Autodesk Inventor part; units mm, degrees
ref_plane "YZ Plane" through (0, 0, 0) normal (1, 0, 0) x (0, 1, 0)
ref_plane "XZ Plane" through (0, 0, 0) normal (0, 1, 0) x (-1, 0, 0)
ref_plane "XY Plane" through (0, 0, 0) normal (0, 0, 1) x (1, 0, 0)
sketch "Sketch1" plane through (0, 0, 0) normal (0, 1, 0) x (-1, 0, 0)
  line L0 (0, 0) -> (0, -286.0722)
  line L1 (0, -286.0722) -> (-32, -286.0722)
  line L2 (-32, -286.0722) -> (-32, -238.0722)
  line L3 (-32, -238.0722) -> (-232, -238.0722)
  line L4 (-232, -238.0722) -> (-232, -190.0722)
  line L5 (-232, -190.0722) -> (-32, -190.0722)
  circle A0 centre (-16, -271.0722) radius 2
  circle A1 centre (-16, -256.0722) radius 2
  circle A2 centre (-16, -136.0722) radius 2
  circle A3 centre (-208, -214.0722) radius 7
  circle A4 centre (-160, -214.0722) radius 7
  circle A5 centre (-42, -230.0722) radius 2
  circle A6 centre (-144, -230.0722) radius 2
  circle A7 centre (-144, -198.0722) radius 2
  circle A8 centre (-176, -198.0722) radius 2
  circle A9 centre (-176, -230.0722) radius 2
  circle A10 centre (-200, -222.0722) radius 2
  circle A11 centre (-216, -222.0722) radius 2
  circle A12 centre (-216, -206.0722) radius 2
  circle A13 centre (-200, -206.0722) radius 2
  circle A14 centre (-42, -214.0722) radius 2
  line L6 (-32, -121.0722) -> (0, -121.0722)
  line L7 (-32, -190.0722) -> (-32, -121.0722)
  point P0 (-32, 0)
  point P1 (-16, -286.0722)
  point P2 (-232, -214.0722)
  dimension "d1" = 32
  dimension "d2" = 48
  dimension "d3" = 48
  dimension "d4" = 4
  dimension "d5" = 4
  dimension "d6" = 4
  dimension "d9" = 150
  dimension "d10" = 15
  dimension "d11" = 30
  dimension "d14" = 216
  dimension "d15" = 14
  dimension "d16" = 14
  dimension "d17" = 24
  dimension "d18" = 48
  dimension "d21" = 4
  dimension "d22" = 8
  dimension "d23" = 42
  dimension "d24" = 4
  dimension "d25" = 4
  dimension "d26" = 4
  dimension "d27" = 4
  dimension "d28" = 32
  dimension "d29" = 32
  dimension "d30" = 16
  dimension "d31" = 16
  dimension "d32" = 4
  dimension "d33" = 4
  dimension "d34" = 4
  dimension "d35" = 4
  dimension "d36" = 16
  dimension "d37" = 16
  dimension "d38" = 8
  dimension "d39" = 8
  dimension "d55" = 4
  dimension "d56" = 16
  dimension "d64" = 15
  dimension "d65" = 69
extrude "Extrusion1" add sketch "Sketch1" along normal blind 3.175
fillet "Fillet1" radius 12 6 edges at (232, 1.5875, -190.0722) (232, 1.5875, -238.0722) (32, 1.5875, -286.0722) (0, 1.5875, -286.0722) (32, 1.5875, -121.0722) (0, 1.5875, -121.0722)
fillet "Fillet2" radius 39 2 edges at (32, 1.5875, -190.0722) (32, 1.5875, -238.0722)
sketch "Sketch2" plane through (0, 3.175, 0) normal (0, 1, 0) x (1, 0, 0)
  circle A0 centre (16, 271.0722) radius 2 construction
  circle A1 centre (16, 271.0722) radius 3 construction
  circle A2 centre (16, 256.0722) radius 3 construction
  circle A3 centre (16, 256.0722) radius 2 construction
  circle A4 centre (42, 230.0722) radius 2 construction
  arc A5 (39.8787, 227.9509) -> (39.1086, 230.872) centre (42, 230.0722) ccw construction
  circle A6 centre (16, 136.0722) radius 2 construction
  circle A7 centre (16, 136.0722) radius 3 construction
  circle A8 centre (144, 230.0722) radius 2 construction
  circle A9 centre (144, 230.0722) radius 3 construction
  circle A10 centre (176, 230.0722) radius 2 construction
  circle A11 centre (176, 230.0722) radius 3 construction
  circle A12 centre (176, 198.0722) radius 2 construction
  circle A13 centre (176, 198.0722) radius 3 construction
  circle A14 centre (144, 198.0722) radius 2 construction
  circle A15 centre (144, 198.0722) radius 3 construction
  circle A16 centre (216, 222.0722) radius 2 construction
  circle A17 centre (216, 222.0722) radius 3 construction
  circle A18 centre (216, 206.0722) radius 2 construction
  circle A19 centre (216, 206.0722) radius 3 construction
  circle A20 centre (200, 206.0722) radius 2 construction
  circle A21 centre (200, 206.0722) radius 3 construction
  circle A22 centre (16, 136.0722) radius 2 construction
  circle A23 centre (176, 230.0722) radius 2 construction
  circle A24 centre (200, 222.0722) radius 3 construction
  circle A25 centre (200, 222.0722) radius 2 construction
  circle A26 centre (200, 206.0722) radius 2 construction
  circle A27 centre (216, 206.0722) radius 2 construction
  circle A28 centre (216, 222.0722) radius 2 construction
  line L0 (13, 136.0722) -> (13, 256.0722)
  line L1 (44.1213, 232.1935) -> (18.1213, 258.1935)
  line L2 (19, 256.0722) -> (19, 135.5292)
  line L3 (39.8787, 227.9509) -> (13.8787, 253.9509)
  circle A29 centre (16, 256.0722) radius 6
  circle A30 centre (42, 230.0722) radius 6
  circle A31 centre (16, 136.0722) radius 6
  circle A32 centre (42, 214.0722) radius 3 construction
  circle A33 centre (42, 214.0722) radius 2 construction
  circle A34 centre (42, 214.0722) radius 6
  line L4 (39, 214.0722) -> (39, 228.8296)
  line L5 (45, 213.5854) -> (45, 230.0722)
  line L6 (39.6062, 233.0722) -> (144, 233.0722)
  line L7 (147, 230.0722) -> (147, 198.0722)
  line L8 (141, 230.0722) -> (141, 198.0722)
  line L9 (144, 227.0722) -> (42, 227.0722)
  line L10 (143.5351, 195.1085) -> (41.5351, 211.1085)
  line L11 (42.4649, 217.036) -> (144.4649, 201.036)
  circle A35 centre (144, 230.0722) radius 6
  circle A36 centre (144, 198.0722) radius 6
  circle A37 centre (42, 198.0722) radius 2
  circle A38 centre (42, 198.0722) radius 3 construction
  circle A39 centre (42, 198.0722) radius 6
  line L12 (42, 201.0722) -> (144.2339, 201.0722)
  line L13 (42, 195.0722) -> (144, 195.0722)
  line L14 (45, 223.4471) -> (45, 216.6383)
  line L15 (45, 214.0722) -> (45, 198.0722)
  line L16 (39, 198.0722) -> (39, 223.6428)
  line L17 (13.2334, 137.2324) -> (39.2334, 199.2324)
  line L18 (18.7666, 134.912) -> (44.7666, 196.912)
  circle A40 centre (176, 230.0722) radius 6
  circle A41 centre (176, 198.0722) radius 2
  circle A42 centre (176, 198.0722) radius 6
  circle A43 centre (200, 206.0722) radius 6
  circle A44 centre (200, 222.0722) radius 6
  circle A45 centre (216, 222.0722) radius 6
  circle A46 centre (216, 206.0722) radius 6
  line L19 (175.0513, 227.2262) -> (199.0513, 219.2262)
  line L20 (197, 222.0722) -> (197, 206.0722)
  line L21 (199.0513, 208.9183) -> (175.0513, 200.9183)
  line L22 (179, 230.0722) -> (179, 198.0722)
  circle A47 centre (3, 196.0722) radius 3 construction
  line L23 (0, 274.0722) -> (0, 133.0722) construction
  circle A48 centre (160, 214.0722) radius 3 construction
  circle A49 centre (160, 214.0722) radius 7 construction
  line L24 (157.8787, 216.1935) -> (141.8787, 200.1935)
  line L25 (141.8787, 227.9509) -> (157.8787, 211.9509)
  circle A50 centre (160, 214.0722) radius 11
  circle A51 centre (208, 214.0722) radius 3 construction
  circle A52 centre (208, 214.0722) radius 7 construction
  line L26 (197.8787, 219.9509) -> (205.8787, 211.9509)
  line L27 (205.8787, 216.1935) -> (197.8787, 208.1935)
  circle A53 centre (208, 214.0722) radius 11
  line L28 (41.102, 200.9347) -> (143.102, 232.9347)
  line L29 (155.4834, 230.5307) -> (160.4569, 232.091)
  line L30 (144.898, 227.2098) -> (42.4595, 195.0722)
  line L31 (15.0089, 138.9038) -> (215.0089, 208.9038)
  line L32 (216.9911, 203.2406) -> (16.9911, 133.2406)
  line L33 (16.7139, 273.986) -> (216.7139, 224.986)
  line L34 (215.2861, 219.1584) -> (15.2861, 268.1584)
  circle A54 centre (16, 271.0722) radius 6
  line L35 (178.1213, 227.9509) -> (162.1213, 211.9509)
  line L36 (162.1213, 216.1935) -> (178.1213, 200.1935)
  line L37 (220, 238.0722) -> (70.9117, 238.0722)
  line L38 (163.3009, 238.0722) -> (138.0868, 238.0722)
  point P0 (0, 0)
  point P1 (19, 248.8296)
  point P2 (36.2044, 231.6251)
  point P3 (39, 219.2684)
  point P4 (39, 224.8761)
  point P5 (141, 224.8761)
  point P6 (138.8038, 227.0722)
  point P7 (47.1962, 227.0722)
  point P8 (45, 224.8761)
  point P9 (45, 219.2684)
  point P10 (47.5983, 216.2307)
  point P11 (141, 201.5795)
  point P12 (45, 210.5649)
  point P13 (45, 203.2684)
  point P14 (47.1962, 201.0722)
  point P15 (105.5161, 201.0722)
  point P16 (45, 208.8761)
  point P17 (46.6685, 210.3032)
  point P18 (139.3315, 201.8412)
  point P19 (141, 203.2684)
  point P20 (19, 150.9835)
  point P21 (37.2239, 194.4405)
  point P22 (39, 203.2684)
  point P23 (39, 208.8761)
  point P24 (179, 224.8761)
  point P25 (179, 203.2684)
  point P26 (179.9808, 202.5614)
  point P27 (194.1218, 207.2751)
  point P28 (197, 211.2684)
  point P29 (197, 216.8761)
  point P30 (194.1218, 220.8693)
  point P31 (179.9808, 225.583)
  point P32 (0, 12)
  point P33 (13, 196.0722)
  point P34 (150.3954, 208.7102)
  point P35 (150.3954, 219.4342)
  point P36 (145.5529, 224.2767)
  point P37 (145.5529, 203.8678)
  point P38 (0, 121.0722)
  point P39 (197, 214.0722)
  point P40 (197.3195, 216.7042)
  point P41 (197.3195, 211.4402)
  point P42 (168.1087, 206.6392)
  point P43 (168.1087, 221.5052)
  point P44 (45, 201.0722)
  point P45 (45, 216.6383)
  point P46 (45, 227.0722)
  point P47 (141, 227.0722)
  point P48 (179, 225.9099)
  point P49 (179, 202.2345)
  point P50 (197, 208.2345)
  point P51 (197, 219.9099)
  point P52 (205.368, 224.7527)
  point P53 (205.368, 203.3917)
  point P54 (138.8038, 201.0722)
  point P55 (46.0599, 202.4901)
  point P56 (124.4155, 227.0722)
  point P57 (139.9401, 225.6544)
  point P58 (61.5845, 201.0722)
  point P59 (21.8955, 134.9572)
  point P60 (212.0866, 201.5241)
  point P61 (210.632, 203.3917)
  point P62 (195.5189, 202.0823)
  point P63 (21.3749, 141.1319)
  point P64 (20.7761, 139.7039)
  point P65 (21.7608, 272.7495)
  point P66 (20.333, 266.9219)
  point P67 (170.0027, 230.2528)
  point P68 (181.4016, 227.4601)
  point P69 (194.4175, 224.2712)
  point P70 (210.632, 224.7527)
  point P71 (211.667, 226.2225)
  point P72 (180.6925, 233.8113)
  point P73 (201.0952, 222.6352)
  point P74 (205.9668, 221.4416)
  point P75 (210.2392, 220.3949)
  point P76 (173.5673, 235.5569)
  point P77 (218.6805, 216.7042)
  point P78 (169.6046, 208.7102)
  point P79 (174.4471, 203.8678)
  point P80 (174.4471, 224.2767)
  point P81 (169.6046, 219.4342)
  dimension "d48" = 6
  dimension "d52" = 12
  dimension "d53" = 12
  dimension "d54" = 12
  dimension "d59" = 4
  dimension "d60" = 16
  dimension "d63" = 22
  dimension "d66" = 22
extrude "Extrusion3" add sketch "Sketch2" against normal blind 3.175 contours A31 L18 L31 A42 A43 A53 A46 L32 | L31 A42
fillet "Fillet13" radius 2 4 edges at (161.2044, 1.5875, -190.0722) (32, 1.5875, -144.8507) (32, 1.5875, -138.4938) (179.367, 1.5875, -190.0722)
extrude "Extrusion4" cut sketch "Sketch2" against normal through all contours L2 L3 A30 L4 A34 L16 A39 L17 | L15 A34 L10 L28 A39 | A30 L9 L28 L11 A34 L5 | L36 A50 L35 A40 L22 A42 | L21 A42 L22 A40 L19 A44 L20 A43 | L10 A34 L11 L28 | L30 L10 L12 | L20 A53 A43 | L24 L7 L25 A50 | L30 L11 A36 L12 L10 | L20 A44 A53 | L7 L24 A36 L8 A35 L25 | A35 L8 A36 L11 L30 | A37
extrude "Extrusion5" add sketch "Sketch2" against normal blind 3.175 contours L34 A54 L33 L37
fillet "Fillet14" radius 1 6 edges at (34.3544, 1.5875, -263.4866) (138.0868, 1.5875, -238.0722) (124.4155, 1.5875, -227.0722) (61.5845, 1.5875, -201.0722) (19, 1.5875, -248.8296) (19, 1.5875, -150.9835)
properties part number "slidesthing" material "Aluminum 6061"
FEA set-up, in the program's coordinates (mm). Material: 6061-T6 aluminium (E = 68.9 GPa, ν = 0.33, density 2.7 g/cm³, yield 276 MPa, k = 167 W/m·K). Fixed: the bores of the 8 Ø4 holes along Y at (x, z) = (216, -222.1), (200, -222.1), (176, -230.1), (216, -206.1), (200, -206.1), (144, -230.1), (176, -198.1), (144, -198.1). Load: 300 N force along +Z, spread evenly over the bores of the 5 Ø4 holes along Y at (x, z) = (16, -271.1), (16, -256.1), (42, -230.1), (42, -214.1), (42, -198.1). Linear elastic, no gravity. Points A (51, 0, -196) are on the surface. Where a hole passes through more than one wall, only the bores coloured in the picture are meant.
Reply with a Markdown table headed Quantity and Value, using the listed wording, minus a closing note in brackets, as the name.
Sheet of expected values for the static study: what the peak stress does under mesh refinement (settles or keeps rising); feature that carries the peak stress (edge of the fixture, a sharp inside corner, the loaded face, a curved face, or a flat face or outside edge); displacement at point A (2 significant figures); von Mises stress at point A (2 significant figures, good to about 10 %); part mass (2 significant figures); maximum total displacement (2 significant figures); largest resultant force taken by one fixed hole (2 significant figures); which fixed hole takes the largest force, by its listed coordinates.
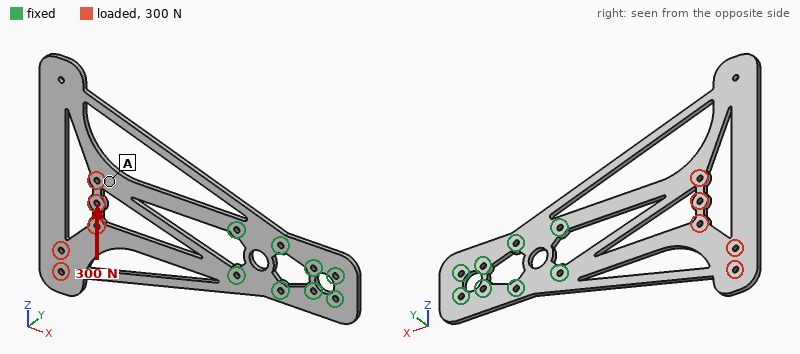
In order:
| Quantity | Value |
|---|---|
| what the peak stress does under mesh refinement | keeps rising |
| feature that carries the peak stress | a sharp inside corner |
| displacement at point A | 0.18 mm |
| von Mises stress at point A | 11 MPa |
| part mass | 110 g |
| maximum total displacement | 0.26 mm |
| largest resultant force taken by one fixed hole | 710 N |
| which fixed hole takes the largest force, by its listed coordinates | (144, -230.1) |
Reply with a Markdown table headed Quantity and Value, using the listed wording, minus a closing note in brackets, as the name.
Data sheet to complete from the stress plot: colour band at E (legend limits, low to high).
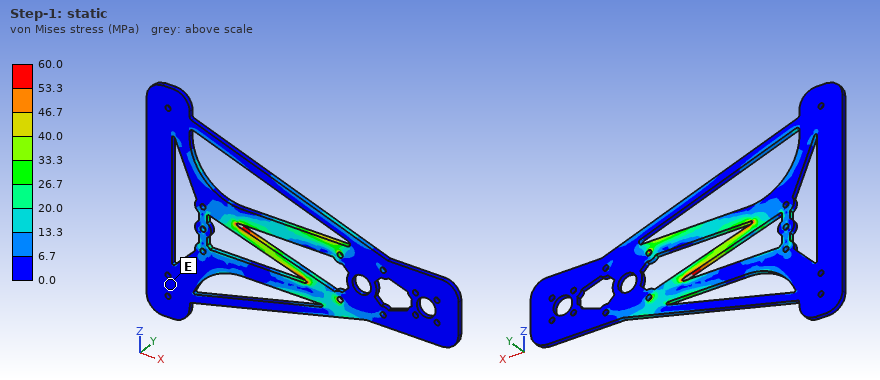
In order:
| Quantity | Value |
|---|---|
| colour band at E | 0.0 to 6.7 MPa |
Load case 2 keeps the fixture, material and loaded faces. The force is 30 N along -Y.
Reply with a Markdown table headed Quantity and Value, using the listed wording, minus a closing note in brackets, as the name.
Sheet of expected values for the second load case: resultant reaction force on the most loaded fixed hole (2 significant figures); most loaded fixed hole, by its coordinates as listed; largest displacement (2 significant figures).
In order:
| Quantity | Value |
|---|---|
| resultant reaction force on the most loaded fixed hole | 29 N |
| most loaded fixed hole, by its coordinates as listed | (144, -230.1) |
| largest displacement | 3.4 mm |
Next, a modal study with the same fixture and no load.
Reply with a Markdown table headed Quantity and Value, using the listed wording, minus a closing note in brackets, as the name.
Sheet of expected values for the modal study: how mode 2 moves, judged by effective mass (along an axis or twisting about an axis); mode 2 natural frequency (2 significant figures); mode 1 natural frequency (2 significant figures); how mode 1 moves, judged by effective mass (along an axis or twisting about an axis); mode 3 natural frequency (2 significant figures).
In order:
| Quantity | Value |
|---|---|
| how mode 2 moves, judged by effective mass | twisting about X |
| mode 2 natural frequency | 150 Hz |
| mode 1 natural frequency | 72 Hz |
| how mode 1 moves, judged by effective mass | along Y |
| mode 3 natural frequency | 570 Hz |
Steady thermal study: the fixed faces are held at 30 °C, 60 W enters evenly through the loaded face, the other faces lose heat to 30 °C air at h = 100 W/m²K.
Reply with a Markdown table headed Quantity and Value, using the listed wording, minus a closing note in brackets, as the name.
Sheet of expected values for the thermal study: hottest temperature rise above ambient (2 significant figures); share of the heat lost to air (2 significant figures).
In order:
| Quantity | Value |
|---|---|
| hottest temperature rise above ambient | 80 K |
| share of the heat lost to air | 93 % |
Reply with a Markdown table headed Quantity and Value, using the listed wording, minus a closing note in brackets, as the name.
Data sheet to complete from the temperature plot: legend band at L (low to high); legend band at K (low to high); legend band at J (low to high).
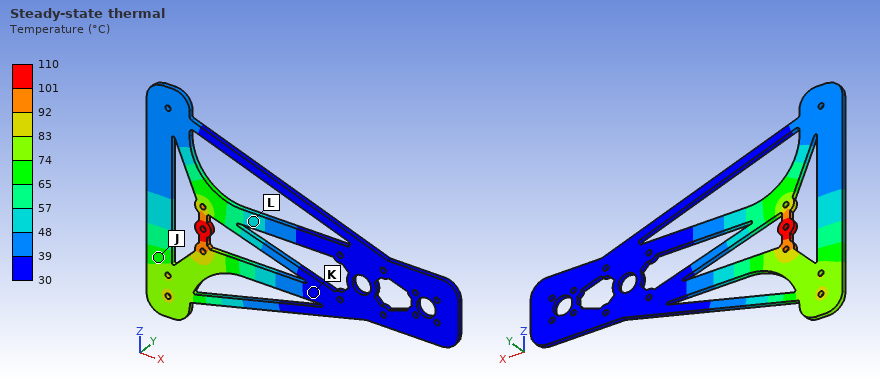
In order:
| Quantity | Value |
|---|---|
| legend band at L | 48 to 57 °C |
| legend band at K | 30 to 39 °C |
| legend band at J | 65 to 74 °C |
